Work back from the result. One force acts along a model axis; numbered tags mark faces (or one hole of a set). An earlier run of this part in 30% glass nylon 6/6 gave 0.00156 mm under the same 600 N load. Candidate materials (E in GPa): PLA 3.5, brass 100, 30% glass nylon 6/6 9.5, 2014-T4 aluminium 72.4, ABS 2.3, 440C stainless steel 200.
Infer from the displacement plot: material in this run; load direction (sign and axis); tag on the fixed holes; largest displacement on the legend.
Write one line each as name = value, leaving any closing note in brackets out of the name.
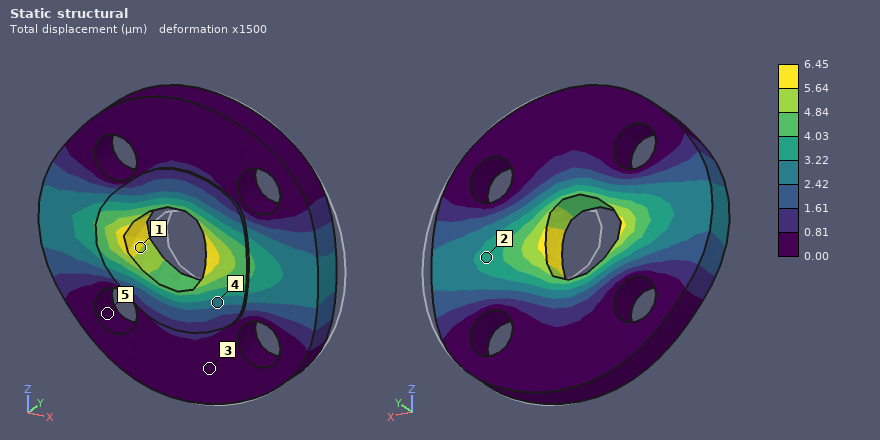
material in this run = ABS
load direction = -X
tag on the fixed holes = 5
largest displacement on the legend = 6.45 µm
